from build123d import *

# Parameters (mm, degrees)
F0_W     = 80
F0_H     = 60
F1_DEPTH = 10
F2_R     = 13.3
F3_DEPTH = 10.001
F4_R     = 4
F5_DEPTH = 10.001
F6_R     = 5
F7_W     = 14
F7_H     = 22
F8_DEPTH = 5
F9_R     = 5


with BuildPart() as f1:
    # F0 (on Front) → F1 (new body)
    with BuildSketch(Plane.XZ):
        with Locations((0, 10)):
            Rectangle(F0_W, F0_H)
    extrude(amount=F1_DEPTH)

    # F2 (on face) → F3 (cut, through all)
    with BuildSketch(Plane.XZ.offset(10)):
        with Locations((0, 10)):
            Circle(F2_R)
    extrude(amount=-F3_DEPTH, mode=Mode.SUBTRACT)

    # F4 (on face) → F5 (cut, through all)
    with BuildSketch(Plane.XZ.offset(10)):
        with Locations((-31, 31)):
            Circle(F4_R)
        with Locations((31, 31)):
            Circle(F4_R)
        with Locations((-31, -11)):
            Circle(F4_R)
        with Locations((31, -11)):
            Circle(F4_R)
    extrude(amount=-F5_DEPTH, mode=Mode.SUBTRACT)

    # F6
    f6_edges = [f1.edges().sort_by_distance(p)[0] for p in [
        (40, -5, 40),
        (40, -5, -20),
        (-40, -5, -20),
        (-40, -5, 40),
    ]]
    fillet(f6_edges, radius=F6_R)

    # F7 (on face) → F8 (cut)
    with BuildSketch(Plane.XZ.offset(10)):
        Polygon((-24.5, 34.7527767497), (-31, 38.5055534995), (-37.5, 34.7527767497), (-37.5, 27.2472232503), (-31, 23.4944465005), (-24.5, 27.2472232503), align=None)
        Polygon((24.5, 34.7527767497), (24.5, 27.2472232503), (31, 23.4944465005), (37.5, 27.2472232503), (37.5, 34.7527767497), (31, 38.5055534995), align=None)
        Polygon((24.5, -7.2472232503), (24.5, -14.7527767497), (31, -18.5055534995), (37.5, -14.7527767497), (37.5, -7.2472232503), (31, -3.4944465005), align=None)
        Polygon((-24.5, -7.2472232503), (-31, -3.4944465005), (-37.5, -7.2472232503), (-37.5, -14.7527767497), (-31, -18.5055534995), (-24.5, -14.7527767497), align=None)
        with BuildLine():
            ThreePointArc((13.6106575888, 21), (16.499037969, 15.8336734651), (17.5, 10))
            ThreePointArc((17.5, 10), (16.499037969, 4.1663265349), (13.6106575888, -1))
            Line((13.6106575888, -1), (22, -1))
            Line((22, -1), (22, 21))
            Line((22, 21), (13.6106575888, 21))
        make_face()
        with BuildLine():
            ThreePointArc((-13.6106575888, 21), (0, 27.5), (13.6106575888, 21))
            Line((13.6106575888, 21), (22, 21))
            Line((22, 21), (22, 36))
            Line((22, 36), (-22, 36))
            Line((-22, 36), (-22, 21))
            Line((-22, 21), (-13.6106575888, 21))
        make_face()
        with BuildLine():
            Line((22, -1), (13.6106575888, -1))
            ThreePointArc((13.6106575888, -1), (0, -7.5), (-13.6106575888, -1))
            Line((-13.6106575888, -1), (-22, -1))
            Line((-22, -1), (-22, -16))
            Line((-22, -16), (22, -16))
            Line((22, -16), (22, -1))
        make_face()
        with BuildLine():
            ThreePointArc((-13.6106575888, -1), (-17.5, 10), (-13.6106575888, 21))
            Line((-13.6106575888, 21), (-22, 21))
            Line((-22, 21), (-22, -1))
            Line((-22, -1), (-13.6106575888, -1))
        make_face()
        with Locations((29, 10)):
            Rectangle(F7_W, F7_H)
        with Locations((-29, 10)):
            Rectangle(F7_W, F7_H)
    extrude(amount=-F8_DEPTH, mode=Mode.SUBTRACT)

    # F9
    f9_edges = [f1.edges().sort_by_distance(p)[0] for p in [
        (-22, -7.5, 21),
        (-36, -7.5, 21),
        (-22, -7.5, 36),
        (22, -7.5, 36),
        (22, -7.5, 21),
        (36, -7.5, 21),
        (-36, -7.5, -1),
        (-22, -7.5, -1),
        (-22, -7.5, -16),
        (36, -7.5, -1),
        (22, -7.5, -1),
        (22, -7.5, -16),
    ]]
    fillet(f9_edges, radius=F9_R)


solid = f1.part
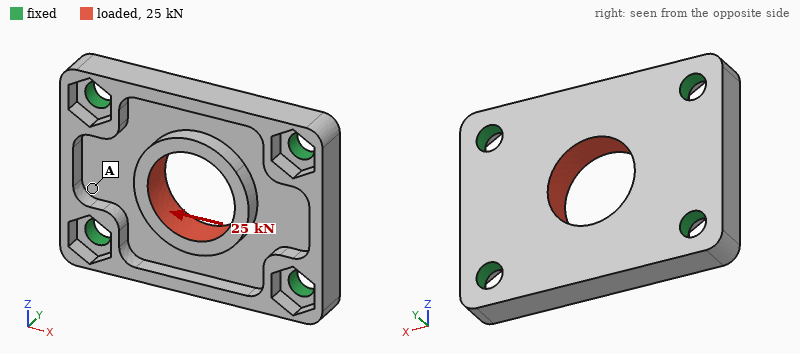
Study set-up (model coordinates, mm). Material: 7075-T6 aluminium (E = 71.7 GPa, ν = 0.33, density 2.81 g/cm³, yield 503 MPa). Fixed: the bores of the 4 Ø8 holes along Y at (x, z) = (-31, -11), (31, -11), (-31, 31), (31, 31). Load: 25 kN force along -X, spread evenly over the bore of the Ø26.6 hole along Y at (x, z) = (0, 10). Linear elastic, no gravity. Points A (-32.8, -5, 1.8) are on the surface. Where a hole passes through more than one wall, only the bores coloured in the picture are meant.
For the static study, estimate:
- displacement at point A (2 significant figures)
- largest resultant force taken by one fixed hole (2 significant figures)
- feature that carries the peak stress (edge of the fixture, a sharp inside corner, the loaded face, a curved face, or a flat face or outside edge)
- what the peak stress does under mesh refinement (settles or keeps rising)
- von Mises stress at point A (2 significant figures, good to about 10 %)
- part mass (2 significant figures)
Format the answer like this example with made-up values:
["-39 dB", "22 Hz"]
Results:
["11 µm", "6.5 kN", "edge of the fixture", "keeps rising", "22 MPa", "81 g"]
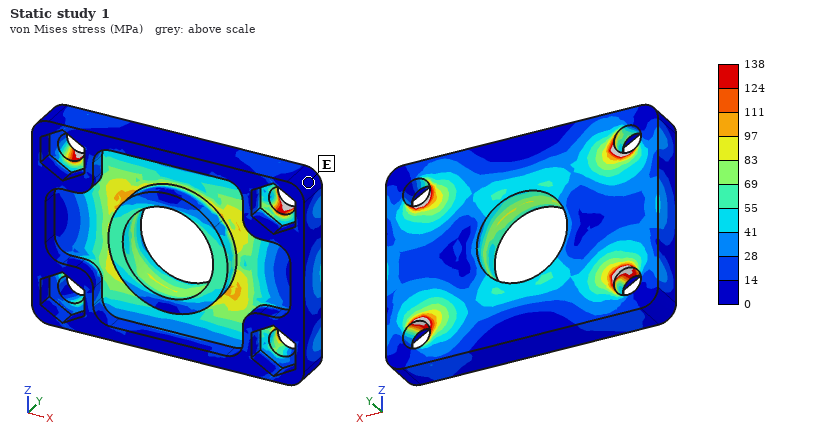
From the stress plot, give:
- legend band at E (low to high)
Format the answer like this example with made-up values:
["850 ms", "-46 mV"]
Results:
["0 to 14 MPa"]
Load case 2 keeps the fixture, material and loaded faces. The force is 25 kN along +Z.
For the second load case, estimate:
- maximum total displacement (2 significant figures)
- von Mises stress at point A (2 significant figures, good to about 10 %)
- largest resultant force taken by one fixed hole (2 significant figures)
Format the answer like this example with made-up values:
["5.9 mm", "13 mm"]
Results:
["78 µm", "40 MPa", "7.1 kN"]
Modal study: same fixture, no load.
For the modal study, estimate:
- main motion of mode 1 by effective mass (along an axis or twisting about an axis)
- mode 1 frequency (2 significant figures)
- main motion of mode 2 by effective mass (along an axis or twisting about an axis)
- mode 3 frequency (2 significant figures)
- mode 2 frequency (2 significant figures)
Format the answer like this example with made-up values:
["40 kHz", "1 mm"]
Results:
["along Y", "9000 Hz", "twisting about X", "14 kHz", "10 kHz"]
